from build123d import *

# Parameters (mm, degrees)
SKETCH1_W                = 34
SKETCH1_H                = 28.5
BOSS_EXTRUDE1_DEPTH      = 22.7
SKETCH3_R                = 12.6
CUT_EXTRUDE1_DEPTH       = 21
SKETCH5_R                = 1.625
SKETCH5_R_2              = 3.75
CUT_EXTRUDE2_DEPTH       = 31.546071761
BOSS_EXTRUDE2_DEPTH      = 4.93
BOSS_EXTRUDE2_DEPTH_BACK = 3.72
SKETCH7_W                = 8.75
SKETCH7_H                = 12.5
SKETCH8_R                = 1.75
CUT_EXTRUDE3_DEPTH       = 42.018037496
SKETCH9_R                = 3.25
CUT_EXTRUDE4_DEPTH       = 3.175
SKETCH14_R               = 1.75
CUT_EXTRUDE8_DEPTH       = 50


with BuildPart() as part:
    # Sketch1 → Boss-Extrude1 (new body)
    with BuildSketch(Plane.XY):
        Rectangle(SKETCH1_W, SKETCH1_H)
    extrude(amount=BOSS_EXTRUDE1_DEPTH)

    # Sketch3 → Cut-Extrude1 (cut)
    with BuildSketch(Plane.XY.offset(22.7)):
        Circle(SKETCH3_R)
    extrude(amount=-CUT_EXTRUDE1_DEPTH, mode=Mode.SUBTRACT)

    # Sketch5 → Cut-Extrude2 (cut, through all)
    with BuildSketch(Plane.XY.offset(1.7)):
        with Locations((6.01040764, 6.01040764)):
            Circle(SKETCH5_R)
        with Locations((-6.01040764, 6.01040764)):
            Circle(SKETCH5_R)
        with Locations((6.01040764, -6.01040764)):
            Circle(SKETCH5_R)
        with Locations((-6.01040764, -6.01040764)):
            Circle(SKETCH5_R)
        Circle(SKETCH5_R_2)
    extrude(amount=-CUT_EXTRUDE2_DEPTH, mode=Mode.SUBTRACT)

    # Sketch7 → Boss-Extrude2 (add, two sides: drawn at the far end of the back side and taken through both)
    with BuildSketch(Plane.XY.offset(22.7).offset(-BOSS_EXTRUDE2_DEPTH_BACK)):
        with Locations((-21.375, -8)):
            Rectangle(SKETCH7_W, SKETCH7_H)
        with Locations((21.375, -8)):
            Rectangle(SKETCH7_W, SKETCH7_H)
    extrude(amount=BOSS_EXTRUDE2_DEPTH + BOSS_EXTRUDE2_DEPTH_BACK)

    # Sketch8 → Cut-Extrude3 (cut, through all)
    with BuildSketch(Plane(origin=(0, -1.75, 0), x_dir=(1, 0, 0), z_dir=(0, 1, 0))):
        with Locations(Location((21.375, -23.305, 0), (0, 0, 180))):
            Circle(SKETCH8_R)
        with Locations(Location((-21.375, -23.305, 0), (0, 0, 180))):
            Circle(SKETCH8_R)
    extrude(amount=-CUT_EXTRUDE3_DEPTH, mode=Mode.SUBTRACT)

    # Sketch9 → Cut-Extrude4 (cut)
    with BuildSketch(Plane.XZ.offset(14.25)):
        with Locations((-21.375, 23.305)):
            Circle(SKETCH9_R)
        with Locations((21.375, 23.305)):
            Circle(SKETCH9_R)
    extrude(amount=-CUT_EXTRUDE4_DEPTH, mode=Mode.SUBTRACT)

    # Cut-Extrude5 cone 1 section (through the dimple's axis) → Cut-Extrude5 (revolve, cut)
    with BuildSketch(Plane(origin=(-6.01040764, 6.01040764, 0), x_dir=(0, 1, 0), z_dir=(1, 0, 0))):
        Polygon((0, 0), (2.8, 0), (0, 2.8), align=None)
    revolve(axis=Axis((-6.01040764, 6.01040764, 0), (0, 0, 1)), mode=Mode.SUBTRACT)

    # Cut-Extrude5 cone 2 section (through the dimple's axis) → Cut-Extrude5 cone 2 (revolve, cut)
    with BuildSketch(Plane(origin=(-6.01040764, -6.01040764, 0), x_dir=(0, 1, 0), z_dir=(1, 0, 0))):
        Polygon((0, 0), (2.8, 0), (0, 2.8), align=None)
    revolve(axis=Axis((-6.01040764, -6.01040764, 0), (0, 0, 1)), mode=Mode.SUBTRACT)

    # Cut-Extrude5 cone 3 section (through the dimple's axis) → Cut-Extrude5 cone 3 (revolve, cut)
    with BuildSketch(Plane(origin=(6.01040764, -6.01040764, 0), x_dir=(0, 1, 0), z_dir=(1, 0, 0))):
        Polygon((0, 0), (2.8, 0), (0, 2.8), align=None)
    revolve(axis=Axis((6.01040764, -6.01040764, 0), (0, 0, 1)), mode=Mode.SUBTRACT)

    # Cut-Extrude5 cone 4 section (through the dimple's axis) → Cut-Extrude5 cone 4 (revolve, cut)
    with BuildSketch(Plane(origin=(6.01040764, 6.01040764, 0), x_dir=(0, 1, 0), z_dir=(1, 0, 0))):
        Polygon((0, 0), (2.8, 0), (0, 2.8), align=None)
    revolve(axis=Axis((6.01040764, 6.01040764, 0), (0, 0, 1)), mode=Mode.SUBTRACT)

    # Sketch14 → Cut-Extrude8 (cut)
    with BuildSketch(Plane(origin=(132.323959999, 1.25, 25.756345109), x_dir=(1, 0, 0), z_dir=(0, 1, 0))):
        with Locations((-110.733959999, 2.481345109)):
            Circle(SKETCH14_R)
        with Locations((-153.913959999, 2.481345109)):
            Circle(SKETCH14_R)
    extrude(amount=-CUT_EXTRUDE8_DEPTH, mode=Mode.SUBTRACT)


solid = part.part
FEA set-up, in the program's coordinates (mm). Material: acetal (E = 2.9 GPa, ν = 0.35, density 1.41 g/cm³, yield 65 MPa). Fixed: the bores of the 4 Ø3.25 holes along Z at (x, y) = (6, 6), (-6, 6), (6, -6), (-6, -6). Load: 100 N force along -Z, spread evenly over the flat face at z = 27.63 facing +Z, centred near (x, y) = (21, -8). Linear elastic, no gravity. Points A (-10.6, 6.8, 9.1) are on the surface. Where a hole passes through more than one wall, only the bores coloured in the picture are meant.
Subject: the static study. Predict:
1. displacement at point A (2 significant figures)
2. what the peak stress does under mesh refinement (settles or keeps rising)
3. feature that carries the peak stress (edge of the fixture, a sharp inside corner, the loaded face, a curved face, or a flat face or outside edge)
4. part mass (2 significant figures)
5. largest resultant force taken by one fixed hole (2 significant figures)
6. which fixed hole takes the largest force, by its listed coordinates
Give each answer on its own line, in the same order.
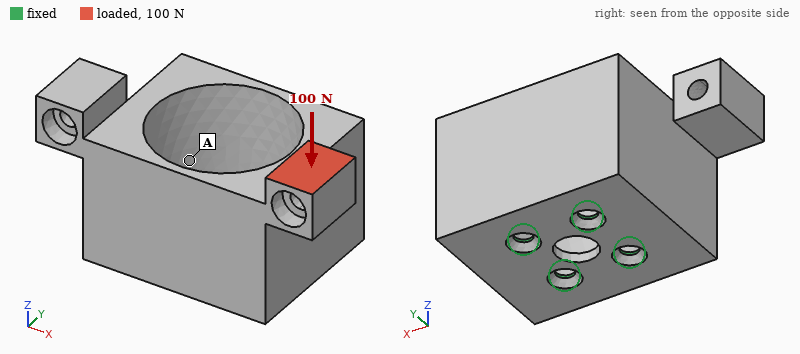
0.14 mm
keeps rising
edge of the fixture
18 g
130 N
(6, -6)
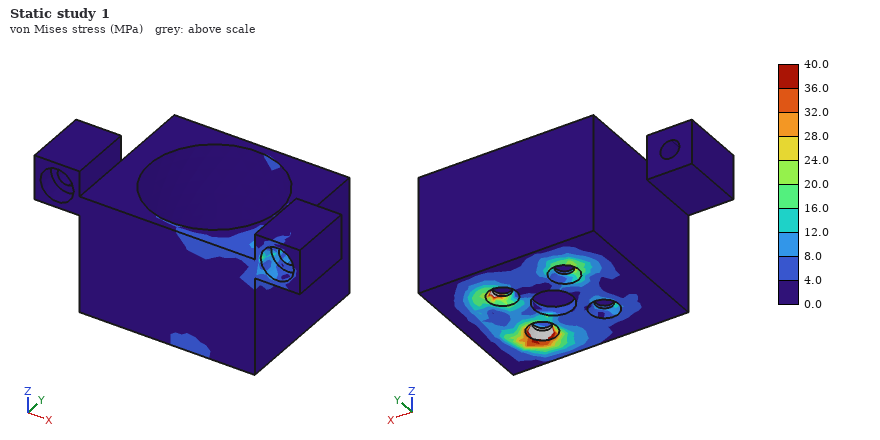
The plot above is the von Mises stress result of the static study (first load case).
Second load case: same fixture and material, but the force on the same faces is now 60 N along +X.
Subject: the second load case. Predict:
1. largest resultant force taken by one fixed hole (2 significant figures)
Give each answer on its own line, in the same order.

61 N
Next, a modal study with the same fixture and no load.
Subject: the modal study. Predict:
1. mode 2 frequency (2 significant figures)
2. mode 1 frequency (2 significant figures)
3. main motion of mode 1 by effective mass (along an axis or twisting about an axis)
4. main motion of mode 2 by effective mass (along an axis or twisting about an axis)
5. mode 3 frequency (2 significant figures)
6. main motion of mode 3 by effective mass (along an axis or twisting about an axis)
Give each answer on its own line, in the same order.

960 Hz
840 Hz
along X
along Y
2200 Hz
along Z
